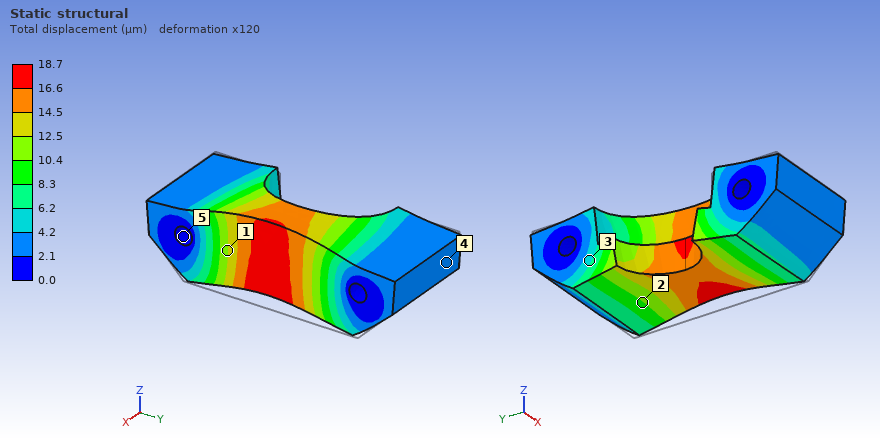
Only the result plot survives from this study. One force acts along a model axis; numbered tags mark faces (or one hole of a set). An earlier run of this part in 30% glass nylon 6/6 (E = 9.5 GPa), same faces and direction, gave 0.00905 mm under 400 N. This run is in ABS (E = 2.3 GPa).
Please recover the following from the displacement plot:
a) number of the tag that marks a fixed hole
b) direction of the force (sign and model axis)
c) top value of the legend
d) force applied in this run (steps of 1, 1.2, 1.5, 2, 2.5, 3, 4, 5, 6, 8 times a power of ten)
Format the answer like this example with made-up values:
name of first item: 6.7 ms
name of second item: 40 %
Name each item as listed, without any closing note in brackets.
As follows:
number of the tag that marks a fixed hole: 5
direction of the force: +Z
top value of the legend: 18.7 µm
force applied in this run: 200 N
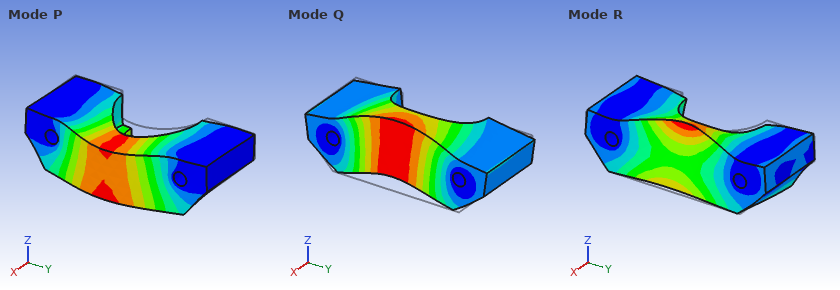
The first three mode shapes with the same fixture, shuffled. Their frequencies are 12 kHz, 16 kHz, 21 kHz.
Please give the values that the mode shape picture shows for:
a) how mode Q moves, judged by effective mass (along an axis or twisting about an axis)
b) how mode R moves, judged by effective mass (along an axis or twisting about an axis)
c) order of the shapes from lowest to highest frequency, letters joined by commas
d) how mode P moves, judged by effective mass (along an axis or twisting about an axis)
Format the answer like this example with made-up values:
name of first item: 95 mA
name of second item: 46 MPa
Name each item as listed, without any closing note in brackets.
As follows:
how mode Q moves, judged by effective mass: along Z
how mode R moves, judged by effective mass: twisting about Y
order of the shapes from lowest to highest frequency, letters joined by commas: Q, P, R
how mode P moves, judged by effective mass: along X
